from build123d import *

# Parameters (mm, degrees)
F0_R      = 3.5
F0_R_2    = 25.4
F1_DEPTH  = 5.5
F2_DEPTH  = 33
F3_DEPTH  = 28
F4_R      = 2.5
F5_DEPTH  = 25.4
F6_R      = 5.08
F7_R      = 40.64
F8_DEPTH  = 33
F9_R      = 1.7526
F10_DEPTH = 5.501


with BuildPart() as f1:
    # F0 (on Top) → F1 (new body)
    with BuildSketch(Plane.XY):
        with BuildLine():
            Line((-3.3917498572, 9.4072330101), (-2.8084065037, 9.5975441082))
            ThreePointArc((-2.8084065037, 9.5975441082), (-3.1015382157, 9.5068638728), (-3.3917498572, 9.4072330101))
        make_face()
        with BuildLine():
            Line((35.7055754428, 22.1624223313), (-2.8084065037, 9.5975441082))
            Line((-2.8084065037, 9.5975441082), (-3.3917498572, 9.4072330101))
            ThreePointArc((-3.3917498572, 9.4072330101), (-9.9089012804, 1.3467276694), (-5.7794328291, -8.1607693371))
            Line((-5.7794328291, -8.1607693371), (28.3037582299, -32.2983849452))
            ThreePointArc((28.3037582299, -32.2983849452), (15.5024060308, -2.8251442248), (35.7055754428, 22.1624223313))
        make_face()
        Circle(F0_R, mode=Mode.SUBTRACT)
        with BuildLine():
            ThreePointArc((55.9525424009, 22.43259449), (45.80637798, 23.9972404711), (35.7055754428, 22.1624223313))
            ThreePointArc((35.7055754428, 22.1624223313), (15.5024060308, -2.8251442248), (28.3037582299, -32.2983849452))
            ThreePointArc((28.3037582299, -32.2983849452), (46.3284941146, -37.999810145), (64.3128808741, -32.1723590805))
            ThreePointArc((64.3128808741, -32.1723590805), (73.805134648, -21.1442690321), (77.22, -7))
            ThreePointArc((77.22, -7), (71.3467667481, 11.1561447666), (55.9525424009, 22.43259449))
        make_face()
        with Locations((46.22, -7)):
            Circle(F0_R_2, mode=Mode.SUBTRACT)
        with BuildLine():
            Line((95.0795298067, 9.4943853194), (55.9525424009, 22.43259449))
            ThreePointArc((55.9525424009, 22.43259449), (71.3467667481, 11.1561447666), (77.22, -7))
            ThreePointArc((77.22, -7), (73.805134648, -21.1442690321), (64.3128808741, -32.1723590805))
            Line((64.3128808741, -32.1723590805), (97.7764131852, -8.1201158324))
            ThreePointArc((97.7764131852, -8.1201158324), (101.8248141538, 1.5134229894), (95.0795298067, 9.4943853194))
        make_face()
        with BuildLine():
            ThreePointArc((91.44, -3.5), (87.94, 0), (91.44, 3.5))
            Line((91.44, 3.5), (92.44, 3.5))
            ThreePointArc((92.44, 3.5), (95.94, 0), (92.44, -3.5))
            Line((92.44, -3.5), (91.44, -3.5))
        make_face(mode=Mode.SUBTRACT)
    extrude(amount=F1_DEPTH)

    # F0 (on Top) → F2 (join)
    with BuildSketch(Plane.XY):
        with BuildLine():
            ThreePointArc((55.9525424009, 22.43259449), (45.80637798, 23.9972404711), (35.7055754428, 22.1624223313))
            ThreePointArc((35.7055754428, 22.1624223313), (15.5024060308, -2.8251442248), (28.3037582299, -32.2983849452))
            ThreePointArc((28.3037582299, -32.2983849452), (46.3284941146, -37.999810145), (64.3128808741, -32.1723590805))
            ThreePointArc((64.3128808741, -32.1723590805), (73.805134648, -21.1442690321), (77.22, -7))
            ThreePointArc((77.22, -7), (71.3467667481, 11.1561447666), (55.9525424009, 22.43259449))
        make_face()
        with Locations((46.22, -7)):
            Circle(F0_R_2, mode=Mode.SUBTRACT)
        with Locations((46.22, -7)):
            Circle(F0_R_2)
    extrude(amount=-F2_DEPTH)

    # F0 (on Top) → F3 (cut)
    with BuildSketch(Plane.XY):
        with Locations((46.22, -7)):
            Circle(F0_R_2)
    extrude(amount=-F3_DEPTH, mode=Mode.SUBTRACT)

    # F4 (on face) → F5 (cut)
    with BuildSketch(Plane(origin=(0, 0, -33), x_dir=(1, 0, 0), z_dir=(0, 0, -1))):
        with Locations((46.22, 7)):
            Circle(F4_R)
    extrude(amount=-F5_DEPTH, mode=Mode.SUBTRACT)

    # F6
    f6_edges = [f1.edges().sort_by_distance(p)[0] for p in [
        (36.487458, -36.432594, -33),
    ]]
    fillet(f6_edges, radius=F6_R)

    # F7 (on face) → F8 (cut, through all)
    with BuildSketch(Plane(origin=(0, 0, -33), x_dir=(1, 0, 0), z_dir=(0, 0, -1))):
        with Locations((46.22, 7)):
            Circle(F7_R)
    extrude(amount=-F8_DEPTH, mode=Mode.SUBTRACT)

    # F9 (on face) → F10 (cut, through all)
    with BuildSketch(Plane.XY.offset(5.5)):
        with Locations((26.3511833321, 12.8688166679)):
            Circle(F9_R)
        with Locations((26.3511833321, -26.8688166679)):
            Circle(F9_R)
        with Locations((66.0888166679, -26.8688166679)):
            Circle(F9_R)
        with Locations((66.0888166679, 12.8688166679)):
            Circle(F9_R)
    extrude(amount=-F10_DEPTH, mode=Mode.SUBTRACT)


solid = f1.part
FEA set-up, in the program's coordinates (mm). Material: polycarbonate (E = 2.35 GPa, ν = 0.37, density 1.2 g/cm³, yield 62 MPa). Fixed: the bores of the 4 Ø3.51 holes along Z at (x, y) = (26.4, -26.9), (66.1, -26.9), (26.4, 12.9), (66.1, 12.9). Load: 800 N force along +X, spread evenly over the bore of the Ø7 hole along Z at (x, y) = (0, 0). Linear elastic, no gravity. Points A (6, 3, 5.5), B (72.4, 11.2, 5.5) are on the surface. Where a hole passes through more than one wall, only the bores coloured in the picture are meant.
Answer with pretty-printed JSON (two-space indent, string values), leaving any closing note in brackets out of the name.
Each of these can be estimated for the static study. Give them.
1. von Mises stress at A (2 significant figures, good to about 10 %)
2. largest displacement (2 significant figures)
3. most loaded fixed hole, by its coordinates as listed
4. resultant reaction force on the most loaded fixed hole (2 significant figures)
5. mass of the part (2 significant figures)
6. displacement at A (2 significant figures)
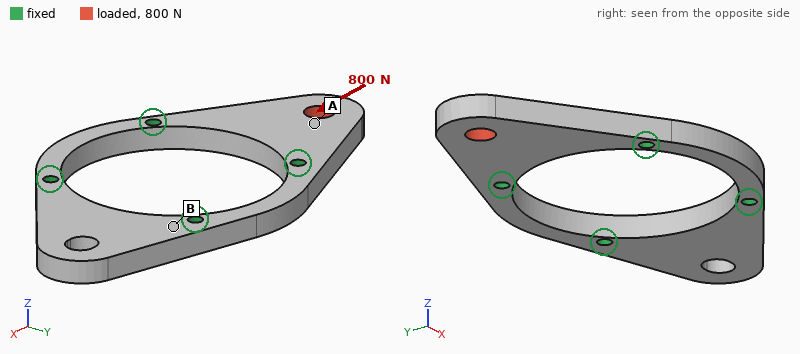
{
  "von Mises stress at A": "6.8 MPa",
  "largest displacement": "0.14 mm",
  "most loaded fixed hole, by its coordinates as listed": "(26.4, 12.9)",
  "resultant reaction force on the most loaded fixed hole": "580 N",
  "mass of the part": "16 g",
  "displacement at A": "0.095 mm"
}
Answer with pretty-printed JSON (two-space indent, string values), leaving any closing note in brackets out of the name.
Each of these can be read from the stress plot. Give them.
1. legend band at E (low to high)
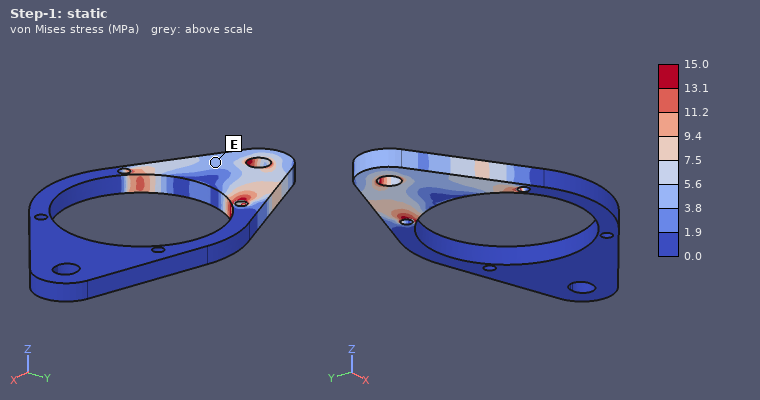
{
  "legend band at E": "3.8 to 5.6 MPa"
}
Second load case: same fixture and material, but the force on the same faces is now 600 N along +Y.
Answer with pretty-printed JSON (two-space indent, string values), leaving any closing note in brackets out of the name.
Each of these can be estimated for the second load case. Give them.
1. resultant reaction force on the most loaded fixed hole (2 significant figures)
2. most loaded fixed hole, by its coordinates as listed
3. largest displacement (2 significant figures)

{
  "resultant reaction force on the most loaded fixed hole": "510 N",
  "most loaded fixed hole, by its coordinates as listed": "(26.4, -26.9)",
  "largest displacement": "0.23 mm"
}
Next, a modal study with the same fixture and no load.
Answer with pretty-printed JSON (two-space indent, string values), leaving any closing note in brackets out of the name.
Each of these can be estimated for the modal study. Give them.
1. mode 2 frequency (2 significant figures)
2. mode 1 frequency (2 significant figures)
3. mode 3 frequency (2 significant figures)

{
  "mode 2 frequency": "960 Hz",
  "mode 1 frequency": "930 Hz",
  "mode 3 frequency": "3300 Hz"
}
